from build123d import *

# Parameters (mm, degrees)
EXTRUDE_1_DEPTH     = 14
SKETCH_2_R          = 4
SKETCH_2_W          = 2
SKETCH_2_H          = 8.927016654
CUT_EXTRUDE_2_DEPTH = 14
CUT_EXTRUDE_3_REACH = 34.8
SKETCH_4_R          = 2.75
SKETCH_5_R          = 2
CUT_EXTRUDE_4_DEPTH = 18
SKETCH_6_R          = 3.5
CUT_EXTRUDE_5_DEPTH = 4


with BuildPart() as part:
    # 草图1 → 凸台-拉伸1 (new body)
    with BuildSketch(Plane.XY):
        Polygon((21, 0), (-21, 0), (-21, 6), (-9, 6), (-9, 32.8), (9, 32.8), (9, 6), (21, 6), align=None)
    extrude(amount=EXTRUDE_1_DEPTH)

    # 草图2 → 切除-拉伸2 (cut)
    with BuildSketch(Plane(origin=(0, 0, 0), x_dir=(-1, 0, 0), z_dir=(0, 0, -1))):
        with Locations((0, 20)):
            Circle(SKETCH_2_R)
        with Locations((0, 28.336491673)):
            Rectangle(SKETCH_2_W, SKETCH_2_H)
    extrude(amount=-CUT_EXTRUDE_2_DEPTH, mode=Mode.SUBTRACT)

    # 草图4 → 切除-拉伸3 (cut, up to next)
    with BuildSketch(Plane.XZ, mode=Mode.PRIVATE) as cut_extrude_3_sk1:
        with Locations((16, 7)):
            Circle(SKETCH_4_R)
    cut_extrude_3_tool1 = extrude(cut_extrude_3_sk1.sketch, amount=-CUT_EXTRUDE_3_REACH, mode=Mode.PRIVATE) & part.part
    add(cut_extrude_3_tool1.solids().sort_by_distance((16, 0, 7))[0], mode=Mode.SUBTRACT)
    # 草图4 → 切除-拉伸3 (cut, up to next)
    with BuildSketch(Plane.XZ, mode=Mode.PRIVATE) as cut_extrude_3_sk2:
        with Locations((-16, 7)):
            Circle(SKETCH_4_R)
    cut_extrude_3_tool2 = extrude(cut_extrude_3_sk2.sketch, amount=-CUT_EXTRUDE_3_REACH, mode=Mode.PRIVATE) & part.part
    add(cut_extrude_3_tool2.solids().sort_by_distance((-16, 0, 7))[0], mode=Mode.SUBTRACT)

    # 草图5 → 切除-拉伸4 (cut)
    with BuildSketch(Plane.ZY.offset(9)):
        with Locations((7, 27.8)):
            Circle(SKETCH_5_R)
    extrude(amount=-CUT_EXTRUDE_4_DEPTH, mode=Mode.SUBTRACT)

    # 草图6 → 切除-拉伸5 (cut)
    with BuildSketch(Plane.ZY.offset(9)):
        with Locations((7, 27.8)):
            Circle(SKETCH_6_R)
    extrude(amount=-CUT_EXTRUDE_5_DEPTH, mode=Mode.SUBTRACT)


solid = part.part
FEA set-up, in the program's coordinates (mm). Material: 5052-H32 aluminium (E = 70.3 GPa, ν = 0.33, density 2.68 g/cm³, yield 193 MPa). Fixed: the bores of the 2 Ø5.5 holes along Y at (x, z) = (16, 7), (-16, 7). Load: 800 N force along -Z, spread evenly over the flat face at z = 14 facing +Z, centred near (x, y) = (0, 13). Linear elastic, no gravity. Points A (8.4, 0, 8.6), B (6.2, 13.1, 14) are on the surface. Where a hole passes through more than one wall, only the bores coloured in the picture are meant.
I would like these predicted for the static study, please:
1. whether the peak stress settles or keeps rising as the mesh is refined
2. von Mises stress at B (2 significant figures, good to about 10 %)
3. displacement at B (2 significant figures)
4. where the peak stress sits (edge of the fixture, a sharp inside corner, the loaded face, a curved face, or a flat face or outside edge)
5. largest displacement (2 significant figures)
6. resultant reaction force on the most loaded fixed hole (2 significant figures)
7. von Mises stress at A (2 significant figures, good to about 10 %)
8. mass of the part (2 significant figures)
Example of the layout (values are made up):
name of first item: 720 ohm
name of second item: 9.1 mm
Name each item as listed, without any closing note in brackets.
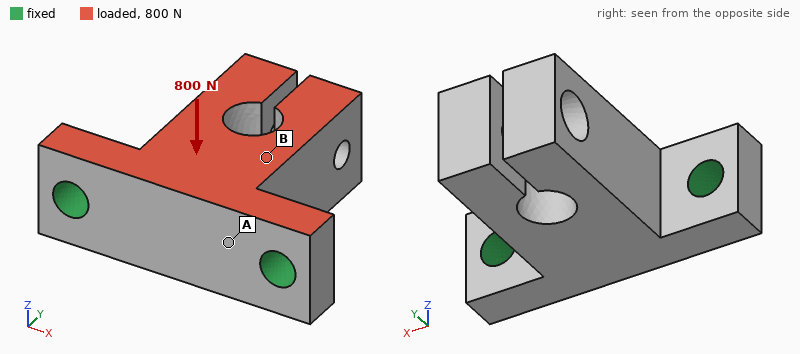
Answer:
whether the peak stress settles or keeps rising as the mesh is refined: keeps rising
von Mises stress at B: 8.1 MPa
displacement at B: 18 µm
where the peak stress sits: edge of the fixture
largest displacement: 47 µm
resultant reaction force on the most loaded fixed hole: 400 N
von Mises stress at A: 17 MPa
mass of the part: 23 g
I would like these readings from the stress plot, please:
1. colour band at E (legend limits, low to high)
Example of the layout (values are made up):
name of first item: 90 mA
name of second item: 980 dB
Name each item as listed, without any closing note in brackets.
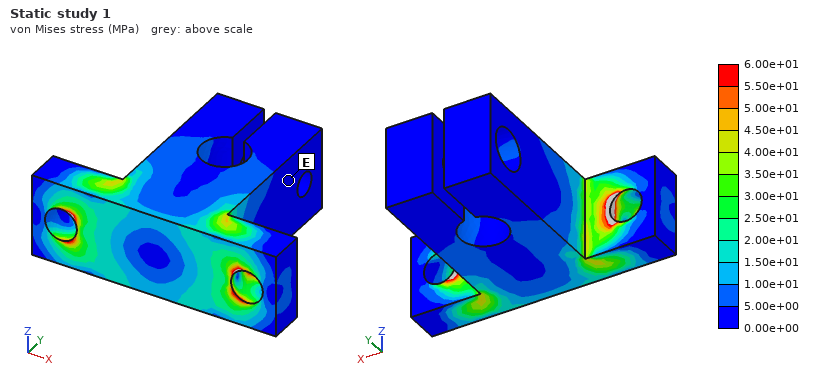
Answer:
colour band at E: 0.00e+00 to 5.00e+00 MPa
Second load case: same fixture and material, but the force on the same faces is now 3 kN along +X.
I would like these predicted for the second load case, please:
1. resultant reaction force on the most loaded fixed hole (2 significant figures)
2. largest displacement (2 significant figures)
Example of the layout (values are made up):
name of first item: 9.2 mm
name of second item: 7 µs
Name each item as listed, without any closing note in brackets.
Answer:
resultant reaction force on the most loaded fixed hole: 2.0 kN
largest displacement: 91 µm
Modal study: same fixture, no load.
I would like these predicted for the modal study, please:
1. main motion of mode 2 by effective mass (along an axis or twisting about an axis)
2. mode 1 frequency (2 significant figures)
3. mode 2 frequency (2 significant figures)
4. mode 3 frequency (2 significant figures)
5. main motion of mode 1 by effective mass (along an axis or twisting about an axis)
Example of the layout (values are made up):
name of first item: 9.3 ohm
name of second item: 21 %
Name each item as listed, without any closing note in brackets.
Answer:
main motion of mode 2 by effective mass: along X
mode 1 frequency: 5300 Hz
mode 2 frequency: 8600 Hz
mode 3 frequency: 11 kHz
main motion of mode 1 by effective mass: along Z
